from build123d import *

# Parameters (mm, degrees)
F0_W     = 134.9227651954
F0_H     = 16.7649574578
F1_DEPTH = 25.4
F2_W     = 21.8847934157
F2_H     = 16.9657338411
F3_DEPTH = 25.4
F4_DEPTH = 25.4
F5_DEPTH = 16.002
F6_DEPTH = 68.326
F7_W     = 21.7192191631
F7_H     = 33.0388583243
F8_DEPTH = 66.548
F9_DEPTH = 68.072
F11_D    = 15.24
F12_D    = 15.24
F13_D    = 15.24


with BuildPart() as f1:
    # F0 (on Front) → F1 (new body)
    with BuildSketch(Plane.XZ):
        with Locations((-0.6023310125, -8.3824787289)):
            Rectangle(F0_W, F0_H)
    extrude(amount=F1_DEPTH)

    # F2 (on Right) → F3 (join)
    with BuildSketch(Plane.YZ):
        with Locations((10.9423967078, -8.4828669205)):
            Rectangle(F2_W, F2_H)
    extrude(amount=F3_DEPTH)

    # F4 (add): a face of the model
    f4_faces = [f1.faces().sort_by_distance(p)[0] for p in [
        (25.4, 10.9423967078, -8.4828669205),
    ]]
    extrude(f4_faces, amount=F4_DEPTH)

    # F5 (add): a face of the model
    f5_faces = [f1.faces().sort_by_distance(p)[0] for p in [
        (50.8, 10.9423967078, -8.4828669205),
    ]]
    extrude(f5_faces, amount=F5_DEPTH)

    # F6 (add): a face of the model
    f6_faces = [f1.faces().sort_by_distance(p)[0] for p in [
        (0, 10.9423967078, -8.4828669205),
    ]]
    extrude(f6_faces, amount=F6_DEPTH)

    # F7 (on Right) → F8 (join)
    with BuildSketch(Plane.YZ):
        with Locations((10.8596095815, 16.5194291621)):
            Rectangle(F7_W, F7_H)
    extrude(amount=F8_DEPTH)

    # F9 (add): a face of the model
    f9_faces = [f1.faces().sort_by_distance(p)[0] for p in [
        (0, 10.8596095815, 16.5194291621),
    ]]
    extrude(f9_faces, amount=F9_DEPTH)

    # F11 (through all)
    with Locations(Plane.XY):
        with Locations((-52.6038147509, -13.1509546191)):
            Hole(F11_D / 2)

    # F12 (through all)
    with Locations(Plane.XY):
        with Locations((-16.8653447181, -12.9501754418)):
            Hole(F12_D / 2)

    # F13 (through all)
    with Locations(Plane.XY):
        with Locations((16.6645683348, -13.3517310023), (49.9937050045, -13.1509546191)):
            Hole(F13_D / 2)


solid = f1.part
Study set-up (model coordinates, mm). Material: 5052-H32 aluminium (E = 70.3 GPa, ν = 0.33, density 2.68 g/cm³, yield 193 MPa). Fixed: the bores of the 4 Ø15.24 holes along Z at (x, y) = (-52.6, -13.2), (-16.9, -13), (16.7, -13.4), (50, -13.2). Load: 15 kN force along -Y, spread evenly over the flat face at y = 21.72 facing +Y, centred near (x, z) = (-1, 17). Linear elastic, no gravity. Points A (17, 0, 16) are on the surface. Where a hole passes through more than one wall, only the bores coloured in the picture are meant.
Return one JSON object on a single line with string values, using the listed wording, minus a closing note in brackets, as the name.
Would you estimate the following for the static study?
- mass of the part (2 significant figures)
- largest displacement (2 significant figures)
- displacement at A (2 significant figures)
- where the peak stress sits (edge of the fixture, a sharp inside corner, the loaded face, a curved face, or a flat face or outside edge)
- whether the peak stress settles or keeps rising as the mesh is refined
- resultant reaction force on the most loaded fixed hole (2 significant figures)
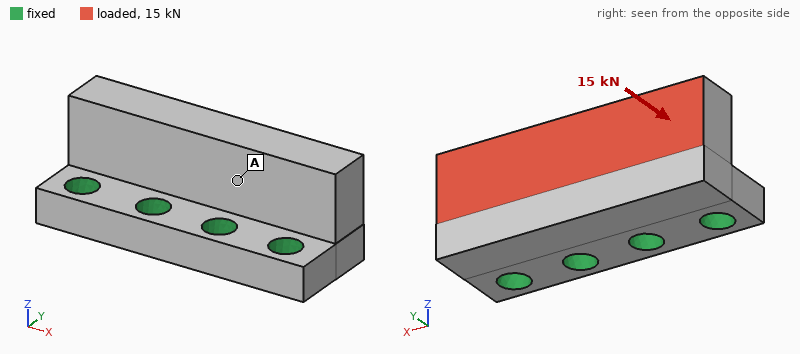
{"mass of the part": "510 g", "largest displacement": "86 µm", "displacement at A": "43 µm", "where the peak stress sits": "edge of the fixture", "whether the peak stress settles or keeps rising as the mesh is refined": "keeps rising", "resultant reaction force on the most loaded fixed hole": "4.1 kN"}
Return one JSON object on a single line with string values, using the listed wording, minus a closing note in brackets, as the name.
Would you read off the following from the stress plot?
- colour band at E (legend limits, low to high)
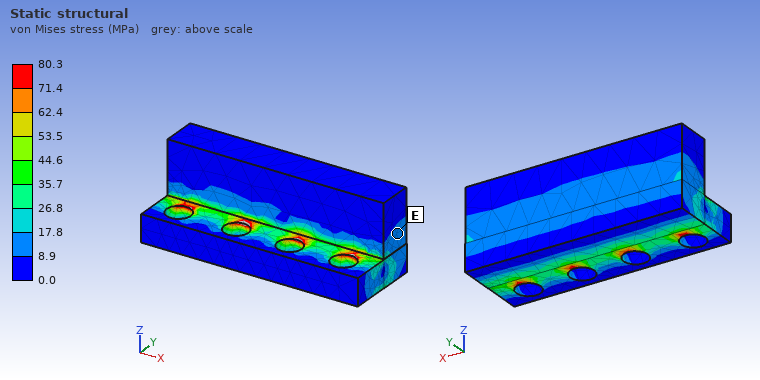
{"colour band at E": "8.9 to 17.8 MPa"}
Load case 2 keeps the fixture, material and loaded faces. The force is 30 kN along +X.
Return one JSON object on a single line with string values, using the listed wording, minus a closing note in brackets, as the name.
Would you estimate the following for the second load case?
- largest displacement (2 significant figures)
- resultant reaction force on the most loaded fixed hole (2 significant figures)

{"largest displacement": "40 µm", "resultant reaction force on the most loaded fixed hole": "12 kN"}
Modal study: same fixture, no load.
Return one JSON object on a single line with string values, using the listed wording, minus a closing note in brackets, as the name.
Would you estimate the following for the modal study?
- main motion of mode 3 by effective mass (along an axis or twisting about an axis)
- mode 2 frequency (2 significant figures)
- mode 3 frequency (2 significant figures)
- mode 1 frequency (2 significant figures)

{"main motion of mode 3 by effective mass": "along X", "mode 2 frequency": "6500 Hz", "mode 3 frequency": "11 kHz", "mode 1 frequency": "4500 Hz"}
